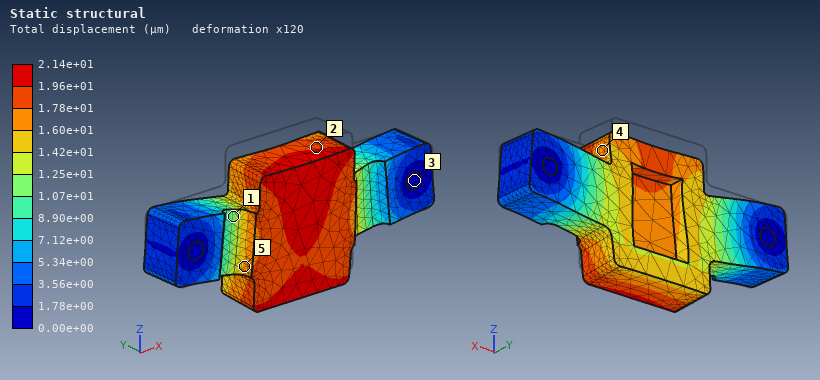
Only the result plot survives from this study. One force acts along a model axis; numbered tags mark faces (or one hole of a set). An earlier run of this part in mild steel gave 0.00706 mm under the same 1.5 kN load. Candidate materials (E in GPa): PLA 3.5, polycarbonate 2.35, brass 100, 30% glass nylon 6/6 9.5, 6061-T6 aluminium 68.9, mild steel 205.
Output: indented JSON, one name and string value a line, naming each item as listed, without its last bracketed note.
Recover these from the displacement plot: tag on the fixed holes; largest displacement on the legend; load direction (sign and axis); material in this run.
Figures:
{
  "tag on the fixed holes": "3",
  "largest displacement on the legend": "2.14e+01 µm",
  "load direction": "-Z",
  "material in this run": "6061-T6 aluminium"
}
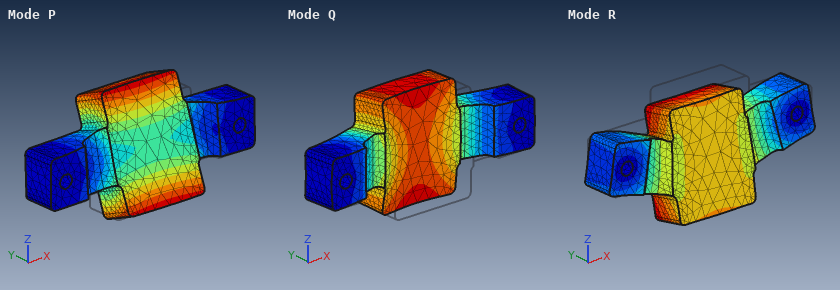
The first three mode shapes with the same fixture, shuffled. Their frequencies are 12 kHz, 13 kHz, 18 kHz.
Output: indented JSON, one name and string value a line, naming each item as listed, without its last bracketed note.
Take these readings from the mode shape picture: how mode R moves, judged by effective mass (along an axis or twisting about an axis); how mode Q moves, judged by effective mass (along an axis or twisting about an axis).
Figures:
{
  "how mode R moves, judged by effective mass": "along Z",
  "how mode Q moves, judged by effective mass": "along Y"
}
